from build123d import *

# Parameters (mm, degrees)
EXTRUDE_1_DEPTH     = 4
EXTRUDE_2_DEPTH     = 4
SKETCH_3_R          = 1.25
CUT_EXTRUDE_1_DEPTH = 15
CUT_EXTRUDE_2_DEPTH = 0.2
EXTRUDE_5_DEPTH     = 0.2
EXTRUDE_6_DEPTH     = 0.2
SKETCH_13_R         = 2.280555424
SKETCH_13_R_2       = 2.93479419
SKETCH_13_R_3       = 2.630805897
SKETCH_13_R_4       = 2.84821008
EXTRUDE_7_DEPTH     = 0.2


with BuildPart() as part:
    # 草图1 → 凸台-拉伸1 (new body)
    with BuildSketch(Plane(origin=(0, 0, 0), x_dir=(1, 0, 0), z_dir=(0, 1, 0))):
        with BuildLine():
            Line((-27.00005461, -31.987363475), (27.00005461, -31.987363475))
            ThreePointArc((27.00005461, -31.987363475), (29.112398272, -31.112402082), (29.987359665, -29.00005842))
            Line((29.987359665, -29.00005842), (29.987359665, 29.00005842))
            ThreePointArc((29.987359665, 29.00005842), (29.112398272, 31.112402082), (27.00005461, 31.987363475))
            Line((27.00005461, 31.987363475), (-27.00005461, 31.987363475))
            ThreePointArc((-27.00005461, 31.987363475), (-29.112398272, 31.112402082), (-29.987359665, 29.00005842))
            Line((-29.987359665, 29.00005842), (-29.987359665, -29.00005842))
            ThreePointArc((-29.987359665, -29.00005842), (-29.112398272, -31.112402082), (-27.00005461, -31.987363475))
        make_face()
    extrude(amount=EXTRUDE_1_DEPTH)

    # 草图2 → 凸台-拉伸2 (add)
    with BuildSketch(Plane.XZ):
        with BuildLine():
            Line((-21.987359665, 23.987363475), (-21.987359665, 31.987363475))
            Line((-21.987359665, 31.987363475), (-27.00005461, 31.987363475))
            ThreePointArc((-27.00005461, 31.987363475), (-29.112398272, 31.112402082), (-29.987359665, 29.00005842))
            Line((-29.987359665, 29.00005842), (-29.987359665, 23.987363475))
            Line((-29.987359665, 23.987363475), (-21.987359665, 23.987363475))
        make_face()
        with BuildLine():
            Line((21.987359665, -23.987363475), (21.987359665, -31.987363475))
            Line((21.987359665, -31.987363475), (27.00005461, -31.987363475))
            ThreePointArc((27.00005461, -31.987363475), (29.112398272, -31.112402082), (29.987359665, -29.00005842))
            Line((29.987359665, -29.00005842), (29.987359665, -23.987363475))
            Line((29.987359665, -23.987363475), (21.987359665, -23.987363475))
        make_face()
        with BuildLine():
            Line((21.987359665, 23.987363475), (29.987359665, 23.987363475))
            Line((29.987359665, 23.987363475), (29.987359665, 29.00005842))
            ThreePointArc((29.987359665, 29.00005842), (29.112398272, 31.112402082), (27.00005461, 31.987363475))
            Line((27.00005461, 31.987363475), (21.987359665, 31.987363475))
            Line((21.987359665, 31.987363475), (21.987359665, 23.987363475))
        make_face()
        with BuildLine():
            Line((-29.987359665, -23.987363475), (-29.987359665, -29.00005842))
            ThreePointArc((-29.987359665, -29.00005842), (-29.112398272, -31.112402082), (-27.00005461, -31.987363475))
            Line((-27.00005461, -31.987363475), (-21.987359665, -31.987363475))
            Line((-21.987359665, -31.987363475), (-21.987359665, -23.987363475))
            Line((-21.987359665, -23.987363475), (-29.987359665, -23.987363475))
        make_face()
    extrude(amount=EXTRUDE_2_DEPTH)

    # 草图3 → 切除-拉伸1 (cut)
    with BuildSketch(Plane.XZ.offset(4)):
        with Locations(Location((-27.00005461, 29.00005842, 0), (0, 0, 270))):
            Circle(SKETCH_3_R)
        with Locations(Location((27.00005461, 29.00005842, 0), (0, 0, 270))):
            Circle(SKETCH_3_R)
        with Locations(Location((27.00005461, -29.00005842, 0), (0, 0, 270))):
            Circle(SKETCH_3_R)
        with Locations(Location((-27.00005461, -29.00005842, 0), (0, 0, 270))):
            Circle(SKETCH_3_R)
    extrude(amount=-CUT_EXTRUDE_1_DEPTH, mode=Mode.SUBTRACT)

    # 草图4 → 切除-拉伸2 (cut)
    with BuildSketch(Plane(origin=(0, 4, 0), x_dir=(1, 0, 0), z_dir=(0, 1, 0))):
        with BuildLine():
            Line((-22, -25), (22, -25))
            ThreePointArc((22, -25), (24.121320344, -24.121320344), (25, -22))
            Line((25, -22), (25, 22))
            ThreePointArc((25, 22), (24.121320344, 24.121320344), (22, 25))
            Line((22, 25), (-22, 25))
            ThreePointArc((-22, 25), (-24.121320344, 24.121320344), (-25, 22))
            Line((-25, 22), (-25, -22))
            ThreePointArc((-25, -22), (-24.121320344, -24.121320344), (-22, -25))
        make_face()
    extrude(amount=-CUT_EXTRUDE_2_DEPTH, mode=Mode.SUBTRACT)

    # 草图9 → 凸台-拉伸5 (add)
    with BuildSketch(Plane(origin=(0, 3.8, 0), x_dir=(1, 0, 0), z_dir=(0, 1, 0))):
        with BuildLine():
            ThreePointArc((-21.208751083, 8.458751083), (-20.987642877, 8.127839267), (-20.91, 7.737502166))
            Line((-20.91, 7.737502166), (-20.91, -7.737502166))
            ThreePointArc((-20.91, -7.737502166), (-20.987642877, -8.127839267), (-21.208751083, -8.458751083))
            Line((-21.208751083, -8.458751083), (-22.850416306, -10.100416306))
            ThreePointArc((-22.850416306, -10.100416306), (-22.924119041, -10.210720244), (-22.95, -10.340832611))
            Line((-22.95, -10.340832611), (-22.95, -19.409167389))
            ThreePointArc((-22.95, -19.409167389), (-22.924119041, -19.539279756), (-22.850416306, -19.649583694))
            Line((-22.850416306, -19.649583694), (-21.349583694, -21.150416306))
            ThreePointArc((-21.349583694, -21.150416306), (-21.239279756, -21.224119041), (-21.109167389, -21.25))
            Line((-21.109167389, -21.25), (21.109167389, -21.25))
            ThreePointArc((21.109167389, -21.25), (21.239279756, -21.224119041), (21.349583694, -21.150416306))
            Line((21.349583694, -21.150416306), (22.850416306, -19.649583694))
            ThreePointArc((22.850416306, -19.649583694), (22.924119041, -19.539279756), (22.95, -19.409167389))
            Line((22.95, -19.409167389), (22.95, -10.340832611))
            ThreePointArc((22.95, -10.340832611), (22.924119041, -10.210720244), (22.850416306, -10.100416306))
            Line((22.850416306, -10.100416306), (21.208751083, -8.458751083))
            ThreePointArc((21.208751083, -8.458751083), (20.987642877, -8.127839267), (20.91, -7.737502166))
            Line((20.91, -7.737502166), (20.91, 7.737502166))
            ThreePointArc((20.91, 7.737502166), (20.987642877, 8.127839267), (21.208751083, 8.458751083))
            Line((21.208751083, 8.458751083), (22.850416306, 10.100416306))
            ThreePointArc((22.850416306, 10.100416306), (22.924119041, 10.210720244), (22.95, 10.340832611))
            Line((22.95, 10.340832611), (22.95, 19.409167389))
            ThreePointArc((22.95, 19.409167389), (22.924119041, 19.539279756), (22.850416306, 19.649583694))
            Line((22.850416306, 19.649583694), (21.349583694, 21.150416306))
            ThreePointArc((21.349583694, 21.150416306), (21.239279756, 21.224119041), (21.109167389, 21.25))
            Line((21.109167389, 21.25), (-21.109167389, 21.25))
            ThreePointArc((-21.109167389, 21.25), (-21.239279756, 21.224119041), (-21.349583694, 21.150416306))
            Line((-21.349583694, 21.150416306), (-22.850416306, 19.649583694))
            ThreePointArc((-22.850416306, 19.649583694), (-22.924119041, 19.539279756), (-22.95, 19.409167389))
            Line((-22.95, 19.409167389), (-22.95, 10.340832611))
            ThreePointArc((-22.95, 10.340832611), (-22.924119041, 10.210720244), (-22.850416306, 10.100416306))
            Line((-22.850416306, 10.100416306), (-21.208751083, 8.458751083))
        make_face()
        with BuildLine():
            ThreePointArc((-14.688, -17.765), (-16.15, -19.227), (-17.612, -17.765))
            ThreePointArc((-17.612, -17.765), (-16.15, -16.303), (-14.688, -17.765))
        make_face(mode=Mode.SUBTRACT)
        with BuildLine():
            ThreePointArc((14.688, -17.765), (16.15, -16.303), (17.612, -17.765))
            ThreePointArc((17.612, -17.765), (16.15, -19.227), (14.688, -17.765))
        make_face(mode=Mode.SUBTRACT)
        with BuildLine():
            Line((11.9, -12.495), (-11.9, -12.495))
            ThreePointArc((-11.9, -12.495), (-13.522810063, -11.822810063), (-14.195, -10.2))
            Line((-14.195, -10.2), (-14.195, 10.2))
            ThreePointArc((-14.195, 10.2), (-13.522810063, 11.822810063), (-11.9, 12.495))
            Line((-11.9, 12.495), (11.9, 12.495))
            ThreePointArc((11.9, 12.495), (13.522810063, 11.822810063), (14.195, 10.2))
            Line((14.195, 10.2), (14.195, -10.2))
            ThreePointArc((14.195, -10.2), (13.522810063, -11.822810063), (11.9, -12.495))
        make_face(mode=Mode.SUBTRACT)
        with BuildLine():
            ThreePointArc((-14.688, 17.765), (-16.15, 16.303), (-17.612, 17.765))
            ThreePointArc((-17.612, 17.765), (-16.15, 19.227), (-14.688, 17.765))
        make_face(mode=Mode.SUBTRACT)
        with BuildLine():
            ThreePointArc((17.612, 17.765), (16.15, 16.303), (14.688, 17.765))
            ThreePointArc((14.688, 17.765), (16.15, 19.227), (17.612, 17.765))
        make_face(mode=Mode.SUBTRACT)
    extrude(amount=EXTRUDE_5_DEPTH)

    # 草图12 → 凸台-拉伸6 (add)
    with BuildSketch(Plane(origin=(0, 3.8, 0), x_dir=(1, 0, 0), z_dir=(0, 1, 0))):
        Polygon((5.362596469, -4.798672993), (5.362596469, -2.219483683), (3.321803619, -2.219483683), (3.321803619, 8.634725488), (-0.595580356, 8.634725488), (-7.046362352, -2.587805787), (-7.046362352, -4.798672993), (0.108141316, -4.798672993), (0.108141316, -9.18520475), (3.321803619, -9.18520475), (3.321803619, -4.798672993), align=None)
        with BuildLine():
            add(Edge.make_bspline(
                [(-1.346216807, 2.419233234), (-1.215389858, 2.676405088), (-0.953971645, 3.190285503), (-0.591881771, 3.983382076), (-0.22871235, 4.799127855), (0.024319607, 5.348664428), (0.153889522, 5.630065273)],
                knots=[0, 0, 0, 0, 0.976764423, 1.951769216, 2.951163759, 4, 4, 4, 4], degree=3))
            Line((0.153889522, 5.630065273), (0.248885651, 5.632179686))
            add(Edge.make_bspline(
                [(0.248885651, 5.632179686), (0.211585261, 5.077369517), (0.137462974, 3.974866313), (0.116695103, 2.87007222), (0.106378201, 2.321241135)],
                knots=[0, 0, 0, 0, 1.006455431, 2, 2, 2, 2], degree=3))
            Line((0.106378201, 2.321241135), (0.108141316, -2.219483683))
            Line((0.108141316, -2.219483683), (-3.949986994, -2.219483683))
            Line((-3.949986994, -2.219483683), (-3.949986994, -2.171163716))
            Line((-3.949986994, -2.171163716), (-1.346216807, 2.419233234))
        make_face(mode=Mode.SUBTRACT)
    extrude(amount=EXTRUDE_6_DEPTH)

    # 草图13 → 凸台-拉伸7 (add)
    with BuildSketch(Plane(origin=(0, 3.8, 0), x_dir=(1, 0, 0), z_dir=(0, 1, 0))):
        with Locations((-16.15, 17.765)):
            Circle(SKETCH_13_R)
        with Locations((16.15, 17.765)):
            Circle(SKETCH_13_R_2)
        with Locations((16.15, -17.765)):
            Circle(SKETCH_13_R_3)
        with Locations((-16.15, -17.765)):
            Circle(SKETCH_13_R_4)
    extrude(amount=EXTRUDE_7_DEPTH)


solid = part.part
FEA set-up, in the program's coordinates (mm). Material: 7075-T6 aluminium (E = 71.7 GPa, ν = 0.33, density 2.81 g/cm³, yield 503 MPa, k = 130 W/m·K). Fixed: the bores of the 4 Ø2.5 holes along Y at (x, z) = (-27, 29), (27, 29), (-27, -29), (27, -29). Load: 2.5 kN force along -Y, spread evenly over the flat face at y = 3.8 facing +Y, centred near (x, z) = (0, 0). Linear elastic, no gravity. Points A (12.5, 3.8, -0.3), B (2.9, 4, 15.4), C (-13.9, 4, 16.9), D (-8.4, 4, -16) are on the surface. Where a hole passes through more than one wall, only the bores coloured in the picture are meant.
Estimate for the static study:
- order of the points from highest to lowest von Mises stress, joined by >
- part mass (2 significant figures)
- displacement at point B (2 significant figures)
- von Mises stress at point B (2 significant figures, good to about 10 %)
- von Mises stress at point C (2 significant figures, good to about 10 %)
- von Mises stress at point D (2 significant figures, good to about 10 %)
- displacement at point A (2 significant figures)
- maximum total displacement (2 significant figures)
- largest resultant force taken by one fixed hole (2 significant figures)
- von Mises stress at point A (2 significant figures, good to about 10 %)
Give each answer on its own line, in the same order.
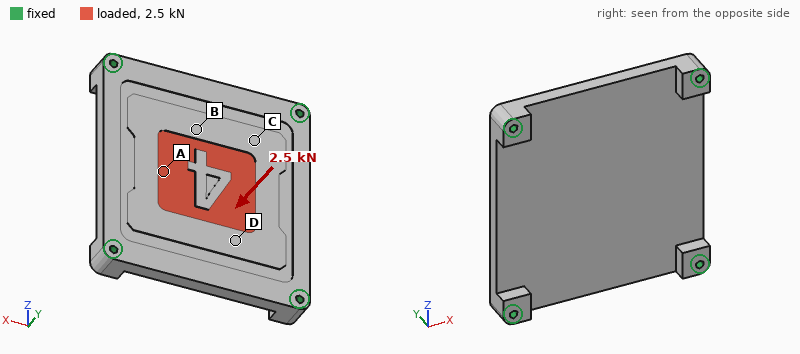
A > B > D > C
45 g
0.14 mm
68 MPa
29 MPa
55 MPa
0.17 mm
0.21 mm
770 N
89 MPa
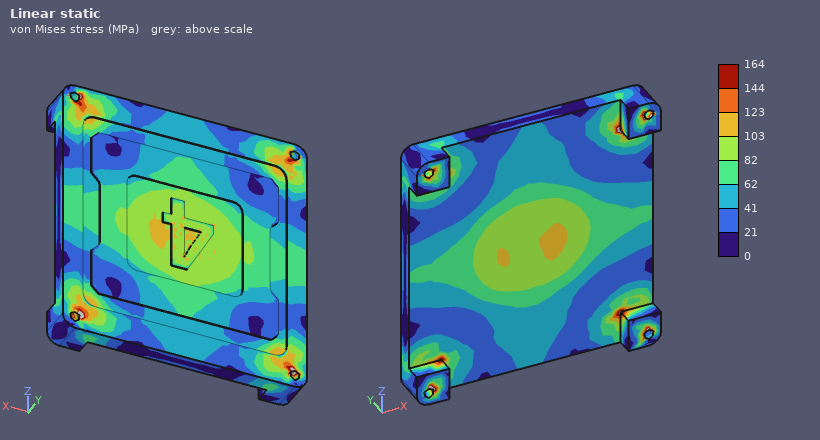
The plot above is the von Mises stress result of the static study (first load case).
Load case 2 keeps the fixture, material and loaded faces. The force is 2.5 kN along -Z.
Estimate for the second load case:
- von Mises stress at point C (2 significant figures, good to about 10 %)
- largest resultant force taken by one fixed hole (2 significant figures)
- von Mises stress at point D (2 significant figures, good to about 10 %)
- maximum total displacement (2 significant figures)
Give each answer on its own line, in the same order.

12 MPa
710 N
11 MPa
8.1 µm
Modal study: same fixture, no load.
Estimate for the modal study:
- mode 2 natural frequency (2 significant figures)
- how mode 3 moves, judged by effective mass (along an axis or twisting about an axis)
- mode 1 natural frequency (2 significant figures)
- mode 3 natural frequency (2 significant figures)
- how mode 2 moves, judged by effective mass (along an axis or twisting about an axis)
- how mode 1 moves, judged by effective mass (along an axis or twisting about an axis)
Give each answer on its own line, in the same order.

7700 Hz
twisting about X
4700 Hz
8400 Hz
twisting about Z
along Y
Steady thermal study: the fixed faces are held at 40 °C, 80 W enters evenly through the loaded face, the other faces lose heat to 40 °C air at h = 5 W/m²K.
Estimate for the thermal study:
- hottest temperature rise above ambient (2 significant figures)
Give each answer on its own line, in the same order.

56 K
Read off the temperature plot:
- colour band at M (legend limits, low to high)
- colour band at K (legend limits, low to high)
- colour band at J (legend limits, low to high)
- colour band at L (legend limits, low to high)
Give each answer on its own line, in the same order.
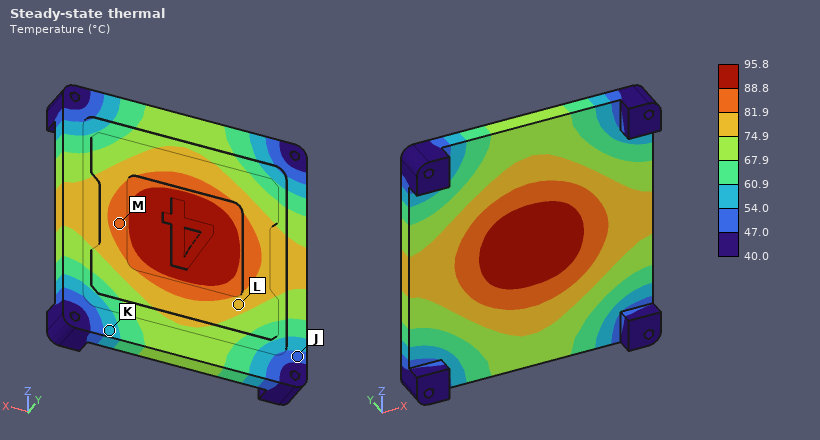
81.9 to 88.8 °C
54.0 to 60.9 °C
47.0 to 54.0 °C
74.9 to 81.9 °C
